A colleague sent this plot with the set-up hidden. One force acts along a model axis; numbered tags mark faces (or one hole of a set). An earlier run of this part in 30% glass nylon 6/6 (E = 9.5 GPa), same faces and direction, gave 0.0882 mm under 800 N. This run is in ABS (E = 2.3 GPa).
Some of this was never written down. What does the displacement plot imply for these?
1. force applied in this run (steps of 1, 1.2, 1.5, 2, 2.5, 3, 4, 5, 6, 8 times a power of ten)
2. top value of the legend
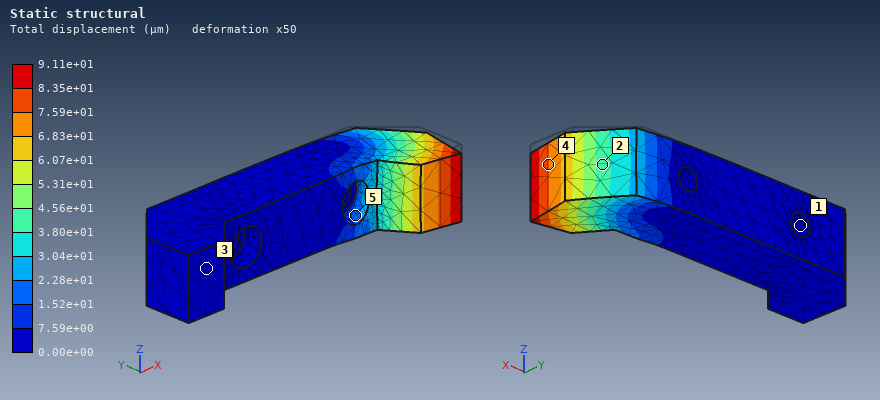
200 N
9.11e+01 µm
